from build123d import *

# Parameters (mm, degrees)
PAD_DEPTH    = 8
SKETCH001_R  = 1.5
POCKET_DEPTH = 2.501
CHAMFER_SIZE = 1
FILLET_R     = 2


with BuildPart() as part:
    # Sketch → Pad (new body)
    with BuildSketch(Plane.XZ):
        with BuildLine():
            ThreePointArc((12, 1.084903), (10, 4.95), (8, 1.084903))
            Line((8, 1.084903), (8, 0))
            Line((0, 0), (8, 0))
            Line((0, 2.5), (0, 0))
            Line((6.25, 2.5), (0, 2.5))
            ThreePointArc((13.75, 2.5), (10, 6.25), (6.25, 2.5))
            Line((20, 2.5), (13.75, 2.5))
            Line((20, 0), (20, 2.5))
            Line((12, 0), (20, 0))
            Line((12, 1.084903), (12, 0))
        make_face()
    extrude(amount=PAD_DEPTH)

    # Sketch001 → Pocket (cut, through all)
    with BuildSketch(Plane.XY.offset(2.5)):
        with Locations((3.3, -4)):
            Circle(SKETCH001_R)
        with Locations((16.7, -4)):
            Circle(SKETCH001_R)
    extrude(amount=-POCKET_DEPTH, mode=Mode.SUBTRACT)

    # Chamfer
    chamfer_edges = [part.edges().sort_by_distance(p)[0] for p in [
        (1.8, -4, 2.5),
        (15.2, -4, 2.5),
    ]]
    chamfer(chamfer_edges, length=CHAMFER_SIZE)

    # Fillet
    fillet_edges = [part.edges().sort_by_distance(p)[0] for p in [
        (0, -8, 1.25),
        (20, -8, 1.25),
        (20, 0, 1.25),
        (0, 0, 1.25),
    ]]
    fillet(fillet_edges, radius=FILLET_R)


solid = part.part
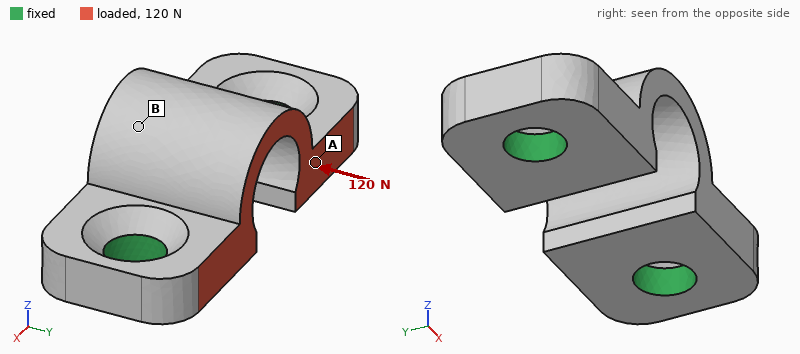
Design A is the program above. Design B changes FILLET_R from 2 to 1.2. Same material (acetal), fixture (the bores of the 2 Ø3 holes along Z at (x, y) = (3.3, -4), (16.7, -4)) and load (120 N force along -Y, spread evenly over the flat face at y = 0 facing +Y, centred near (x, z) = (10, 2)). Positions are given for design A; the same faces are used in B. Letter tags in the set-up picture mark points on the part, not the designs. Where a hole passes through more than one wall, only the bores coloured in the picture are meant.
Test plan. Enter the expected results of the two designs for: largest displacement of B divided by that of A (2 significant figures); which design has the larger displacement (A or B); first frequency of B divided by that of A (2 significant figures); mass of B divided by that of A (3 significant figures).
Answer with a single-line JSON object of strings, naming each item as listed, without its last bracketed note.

{"largest displacement of B divided by that of A": "0.91", "which design has the larger displacement": "A", "first frequency of B divided by that of A": "1.00", "mass of B divided by that of A": "1.02"}
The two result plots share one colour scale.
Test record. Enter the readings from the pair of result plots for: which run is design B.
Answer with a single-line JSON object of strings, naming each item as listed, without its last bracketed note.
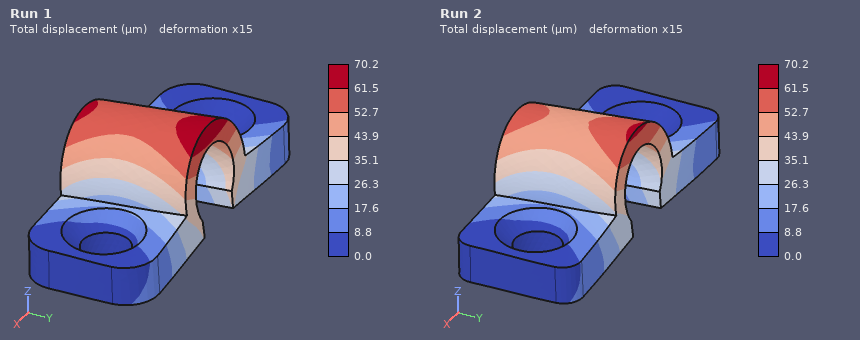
{"which run is design B": "Run 2"}
